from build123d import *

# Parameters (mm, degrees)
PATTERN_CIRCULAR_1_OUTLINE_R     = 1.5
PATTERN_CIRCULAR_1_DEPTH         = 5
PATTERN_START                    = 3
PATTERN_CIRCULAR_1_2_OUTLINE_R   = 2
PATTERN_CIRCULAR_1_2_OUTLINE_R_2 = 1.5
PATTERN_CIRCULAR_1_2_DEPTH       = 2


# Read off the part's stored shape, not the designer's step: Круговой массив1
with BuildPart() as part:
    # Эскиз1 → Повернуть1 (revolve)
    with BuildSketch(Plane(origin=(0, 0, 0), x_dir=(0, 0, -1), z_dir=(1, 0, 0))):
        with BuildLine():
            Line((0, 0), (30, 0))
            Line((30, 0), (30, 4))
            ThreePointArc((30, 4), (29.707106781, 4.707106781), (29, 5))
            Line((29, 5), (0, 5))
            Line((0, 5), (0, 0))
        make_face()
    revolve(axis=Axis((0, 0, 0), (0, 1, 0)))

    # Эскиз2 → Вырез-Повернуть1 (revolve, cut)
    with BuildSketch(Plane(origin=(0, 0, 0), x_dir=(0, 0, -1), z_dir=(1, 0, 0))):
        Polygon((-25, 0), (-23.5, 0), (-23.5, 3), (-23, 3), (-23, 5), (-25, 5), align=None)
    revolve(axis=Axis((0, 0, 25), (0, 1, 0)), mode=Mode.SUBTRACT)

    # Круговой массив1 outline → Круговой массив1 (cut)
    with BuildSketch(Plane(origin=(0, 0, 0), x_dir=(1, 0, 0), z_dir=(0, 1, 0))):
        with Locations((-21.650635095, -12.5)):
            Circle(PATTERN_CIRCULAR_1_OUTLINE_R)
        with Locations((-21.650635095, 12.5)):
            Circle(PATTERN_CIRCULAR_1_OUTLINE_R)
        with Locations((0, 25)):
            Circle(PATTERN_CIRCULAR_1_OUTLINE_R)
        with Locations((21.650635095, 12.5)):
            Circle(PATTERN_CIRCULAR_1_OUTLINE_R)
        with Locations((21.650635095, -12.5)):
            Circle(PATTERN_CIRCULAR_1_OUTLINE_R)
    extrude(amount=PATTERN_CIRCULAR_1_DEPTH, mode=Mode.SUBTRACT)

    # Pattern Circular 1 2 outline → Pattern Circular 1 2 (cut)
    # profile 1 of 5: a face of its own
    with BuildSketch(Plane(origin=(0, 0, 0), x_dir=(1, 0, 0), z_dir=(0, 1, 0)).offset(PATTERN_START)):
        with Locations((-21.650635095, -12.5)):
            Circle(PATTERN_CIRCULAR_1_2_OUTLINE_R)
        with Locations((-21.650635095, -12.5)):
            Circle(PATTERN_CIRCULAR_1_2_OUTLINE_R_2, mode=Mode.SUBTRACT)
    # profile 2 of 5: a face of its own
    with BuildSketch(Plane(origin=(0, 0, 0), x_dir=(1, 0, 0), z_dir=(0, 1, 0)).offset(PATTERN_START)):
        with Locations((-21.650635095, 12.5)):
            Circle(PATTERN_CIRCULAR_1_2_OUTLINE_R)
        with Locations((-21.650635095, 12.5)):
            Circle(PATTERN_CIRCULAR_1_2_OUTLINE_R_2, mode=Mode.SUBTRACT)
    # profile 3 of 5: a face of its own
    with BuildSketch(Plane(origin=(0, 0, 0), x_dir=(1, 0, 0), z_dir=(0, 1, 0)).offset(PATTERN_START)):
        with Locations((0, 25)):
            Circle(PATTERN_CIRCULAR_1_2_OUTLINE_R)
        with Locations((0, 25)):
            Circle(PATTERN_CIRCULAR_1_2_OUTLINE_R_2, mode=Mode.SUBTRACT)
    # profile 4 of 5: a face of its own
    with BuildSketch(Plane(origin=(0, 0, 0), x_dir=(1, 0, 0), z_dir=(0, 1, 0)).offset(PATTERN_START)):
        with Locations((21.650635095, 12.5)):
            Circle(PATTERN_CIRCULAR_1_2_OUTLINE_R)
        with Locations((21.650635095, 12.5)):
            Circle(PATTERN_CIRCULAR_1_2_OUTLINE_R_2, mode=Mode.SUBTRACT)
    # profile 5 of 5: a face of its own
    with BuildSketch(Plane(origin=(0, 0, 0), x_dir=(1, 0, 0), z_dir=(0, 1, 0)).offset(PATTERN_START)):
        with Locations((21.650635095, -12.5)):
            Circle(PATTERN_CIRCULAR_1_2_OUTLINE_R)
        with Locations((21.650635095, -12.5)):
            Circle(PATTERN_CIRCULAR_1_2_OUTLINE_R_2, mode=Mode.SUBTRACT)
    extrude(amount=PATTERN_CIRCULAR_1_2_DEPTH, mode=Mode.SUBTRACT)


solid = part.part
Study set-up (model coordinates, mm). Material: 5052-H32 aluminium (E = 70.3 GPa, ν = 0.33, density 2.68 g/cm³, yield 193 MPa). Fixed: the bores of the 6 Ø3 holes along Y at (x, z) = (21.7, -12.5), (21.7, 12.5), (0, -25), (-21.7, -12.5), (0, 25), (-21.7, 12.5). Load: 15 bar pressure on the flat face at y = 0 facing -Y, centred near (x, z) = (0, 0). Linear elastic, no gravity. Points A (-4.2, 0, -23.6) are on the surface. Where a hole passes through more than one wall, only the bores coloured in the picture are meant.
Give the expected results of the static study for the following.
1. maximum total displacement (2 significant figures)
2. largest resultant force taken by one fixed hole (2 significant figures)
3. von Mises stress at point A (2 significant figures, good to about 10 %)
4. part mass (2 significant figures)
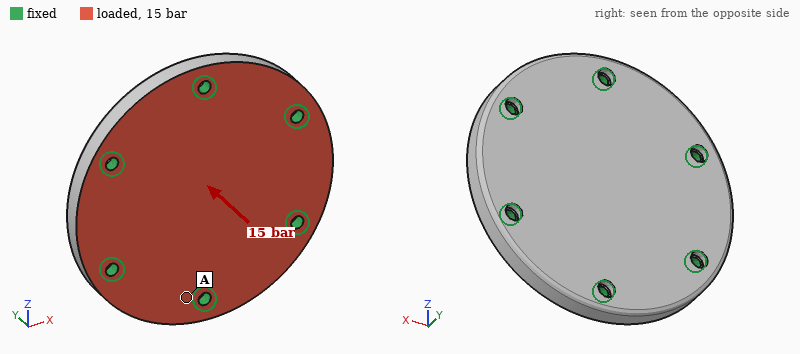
23 µm
730 N
16 MPa
37 g
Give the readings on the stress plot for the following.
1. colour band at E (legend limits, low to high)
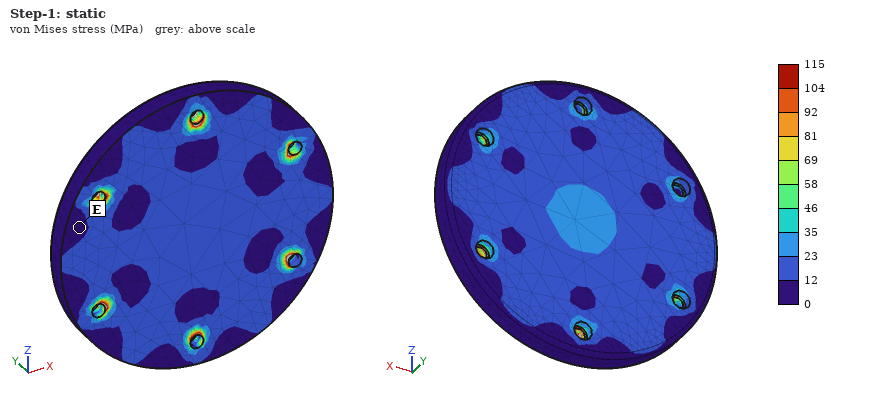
0 to 12 MPa
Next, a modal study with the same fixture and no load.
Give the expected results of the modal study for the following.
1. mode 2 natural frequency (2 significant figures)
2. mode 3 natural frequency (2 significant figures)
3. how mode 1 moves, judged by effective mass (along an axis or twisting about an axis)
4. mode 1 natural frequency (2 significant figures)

24 kHz
25 kHz
along Y
13 kHz
